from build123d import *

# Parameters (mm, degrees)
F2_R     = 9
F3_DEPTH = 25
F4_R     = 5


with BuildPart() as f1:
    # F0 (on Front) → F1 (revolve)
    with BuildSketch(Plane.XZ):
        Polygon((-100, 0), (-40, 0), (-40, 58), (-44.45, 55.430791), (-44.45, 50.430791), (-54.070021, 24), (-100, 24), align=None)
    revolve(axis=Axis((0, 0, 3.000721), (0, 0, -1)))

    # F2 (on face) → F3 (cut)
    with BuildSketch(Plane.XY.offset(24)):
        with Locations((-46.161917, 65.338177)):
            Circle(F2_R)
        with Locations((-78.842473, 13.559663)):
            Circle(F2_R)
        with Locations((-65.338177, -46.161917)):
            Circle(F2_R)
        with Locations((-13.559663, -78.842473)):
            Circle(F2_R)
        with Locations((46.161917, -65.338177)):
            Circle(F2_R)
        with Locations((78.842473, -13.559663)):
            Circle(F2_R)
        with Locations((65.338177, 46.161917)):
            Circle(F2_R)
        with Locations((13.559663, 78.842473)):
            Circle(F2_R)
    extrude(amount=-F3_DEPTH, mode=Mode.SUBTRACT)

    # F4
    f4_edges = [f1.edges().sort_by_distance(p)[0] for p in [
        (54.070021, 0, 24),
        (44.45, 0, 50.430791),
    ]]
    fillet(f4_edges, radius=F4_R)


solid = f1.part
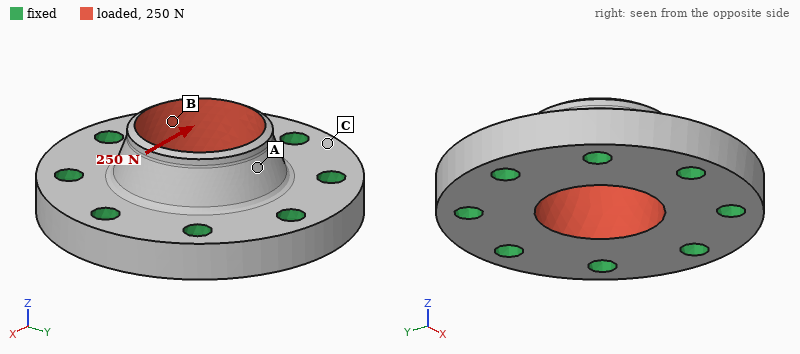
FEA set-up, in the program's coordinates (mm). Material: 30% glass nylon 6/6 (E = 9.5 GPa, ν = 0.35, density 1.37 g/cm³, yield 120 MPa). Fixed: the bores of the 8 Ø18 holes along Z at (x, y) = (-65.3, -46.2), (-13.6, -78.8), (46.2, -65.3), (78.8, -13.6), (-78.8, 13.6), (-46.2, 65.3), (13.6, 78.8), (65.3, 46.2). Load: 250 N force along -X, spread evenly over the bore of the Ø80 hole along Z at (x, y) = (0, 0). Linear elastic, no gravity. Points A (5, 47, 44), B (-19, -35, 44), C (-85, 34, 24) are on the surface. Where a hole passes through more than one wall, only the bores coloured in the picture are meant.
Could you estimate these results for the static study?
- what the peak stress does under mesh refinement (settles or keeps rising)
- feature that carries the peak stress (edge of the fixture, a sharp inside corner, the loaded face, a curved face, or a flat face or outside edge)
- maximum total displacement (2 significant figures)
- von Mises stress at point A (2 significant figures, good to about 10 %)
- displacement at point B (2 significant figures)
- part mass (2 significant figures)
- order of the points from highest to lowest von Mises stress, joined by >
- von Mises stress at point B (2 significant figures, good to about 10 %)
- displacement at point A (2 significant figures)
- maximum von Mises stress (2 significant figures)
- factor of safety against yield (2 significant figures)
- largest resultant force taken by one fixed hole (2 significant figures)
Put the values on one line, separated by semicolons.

settles; the loaded face; 1.6 µm; 0.070 MPa; 0.64 µm; 910 g; B > A > C; 0.12 MPa; 0.48 µm; 0.22 MPa; 540; 48 N
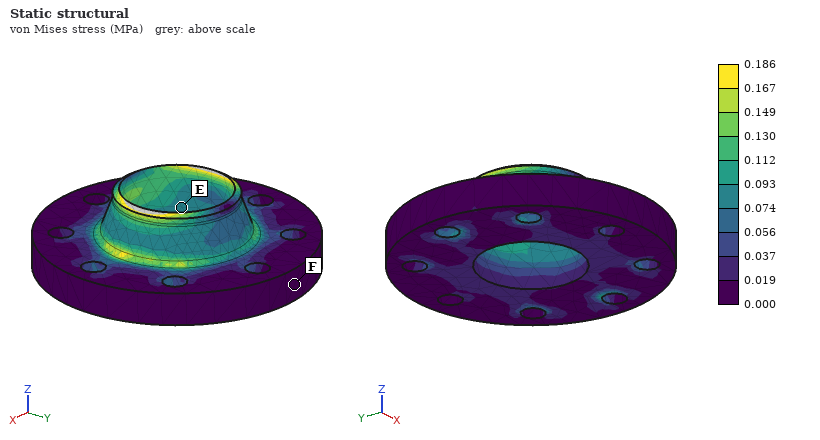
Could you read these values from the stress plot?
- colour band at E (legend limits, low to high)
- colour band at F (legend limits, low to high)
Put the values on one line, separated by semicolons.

0.074 to 0.093 MPa; 0.000 to 0.019 MPa
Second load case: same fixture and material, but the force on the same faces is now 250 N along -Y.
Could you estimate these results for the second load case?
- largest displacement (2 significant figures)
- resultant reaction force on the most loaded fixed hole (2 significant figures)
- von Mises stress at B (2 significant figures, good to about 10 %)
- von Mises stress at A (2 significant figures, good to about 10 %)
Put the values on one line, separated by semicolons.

1.6 µm; 48 N; 0.096 MPa; 0.096 MPa
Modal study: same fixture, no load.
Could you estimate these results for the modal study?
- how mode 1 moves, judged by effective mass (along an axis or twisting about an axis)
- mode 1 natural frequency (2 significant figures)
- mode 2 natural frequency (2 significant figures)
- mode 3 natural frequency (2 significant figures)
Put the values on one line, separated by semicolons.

along Z; 6000 Hz; 7100 Hz; 7100 Hz
